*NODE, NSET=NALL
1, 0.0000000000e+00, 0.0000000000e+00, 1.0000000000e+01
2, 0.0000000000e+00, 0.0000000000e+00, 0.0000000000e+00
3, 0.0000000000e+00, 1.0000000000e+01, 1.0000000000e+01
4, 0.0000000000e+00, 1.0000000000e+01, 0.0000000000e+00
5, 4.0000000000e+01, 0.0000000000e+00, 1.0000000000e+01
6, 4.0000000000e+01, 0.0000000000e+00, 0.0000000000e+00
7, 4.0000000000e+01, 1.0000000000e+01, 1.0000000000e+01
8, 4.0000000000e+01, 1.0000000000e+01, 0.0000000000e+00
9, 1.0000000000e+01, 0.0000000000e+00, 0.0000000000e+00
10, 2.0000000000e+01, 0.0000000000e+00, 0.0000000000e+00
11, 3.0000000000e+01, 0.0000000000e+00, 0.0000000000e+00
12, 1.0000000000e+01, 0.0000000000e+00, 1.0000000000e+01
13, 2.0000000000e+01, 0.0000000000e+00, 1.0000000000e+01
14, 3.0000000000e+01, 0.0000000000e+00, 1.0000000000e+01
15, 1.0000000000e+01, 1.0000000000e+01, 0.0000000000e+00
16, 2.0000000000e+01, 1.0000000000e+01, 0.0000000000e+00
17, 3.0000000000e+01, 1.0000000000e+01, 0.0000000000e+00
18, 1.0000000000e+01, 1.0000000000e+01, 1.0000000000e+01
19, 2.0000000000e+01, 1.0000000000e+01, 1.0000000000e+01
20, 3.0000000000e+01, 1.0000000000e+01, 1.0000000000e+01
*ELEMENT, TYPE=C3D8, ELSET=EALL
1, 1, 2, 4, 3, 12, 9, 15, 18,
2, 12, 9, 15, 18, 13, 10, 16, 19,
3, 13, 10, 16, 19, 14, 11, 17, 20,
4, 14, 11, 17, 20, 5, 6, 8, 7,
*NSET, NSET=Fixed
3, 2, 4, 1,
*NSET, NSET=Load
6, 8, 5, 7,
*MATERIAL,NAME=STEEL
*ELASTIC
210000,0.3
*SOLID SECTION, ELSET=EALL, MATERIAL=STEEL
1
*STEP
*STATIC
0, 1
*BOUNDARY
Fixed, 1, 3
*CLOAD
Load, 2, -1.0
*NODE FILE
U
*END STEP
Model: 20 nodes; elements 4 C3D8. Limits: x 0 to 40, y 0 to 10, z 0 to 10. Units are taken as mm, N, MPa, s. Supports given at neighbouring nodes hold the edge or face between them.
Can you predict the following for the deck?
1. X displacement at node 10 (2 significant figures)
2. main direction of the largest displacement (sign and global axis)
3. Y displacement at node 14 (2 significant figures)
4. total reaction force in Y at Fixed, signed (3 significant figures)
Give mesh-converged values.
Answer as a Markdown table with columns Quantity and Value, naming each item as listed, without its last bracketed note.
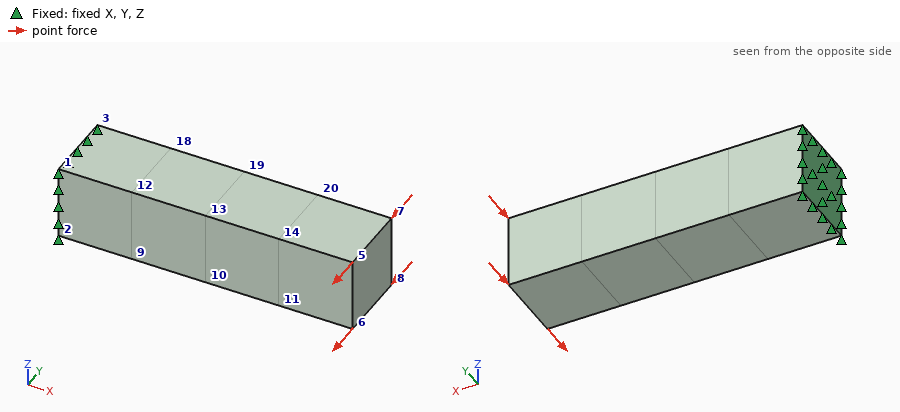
| Quantity | Value |
|---|---|
| X displacement at node 10 | -6.7e-05 mm |
| main direction of the largest displacement | -Y |
| Y displacement at node 14 | -3.2e-04 mm |
| total reaction force in Y at Fixed, signed | 4.00 N |
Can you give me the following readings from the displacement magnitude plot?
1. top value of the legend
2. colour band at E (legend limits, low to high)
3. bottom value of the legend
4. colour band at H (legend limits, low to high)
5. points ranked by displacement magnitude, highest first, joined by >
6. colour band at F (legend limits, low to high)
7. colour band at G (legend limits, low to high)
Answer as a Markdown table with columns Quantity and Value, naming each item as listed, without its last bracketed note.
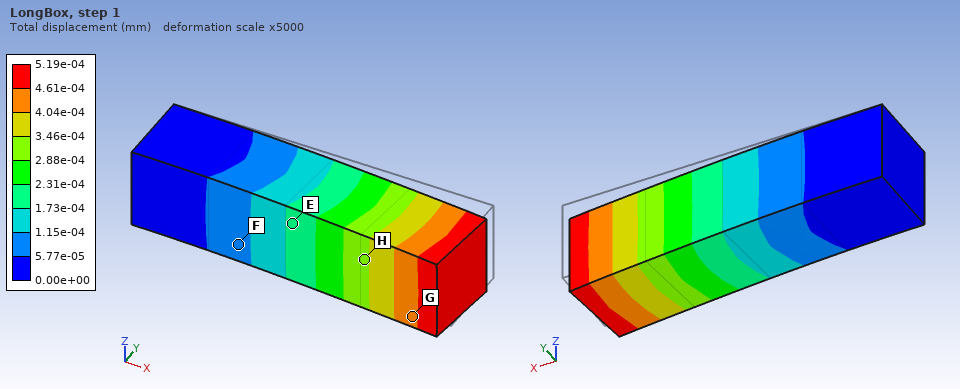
| Quantity | Value |
|---|---|
| top value of the legend | 5.19e-04 mm |
| colour band at E | 1.73e-04 to 2.31e-04 mm |
| bottom value of the legend | 0.00e+00 mm |
| colour band at H | 2.88e-04 to 3.46e-04 mm |
| points ranked by displacement magnitude, highest first, joined by > | G > H > E > F |
| colour band at F | 5.77e-05 to 1.15e-04 mm |
| colour band at G | 4.04e-04 to 4.61e-04 mm |
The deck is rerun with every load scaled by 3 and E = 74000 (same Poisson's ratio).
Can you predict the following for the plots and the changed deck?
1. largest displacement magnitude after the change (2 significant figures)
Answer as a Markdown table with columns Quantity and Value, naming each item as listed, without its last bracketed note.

| Quantity | Value |
|---|---|
| largest displacement magnitude after the change | 0.0044 mm |
